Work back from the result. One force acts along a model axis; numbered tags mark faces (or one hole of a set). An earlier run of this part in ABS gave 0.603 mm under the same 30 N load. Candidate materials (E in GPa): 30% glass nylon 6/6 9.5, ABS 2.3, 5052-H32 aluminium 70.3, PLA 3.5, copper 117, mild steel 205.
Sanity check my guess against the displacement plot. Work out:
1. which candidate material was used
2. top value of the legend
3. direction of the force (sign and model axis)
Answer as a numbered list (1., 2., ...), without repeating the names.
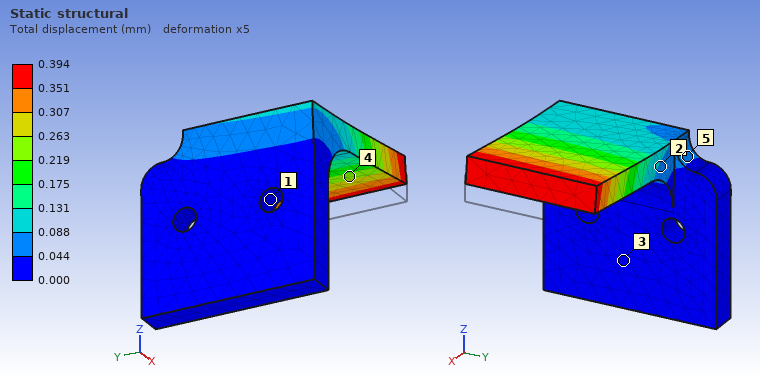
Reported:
1. PLA
2. 0.394 mm
3. +Z
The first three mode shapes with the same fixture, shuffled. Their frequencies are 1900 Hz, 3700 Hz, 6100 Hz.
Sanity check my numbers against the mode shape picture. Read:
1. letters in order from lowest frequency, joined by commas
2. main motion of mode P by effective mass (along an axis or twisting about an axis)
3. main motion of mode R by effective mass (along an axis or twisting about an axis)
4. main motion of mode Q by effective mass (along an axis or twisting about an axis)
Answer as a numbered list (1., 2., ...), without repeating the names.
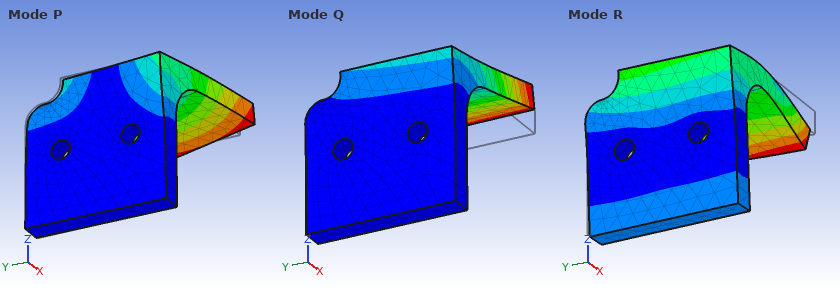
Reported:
1. Q, P, R
2. along Y
3. along X
4. along Z
